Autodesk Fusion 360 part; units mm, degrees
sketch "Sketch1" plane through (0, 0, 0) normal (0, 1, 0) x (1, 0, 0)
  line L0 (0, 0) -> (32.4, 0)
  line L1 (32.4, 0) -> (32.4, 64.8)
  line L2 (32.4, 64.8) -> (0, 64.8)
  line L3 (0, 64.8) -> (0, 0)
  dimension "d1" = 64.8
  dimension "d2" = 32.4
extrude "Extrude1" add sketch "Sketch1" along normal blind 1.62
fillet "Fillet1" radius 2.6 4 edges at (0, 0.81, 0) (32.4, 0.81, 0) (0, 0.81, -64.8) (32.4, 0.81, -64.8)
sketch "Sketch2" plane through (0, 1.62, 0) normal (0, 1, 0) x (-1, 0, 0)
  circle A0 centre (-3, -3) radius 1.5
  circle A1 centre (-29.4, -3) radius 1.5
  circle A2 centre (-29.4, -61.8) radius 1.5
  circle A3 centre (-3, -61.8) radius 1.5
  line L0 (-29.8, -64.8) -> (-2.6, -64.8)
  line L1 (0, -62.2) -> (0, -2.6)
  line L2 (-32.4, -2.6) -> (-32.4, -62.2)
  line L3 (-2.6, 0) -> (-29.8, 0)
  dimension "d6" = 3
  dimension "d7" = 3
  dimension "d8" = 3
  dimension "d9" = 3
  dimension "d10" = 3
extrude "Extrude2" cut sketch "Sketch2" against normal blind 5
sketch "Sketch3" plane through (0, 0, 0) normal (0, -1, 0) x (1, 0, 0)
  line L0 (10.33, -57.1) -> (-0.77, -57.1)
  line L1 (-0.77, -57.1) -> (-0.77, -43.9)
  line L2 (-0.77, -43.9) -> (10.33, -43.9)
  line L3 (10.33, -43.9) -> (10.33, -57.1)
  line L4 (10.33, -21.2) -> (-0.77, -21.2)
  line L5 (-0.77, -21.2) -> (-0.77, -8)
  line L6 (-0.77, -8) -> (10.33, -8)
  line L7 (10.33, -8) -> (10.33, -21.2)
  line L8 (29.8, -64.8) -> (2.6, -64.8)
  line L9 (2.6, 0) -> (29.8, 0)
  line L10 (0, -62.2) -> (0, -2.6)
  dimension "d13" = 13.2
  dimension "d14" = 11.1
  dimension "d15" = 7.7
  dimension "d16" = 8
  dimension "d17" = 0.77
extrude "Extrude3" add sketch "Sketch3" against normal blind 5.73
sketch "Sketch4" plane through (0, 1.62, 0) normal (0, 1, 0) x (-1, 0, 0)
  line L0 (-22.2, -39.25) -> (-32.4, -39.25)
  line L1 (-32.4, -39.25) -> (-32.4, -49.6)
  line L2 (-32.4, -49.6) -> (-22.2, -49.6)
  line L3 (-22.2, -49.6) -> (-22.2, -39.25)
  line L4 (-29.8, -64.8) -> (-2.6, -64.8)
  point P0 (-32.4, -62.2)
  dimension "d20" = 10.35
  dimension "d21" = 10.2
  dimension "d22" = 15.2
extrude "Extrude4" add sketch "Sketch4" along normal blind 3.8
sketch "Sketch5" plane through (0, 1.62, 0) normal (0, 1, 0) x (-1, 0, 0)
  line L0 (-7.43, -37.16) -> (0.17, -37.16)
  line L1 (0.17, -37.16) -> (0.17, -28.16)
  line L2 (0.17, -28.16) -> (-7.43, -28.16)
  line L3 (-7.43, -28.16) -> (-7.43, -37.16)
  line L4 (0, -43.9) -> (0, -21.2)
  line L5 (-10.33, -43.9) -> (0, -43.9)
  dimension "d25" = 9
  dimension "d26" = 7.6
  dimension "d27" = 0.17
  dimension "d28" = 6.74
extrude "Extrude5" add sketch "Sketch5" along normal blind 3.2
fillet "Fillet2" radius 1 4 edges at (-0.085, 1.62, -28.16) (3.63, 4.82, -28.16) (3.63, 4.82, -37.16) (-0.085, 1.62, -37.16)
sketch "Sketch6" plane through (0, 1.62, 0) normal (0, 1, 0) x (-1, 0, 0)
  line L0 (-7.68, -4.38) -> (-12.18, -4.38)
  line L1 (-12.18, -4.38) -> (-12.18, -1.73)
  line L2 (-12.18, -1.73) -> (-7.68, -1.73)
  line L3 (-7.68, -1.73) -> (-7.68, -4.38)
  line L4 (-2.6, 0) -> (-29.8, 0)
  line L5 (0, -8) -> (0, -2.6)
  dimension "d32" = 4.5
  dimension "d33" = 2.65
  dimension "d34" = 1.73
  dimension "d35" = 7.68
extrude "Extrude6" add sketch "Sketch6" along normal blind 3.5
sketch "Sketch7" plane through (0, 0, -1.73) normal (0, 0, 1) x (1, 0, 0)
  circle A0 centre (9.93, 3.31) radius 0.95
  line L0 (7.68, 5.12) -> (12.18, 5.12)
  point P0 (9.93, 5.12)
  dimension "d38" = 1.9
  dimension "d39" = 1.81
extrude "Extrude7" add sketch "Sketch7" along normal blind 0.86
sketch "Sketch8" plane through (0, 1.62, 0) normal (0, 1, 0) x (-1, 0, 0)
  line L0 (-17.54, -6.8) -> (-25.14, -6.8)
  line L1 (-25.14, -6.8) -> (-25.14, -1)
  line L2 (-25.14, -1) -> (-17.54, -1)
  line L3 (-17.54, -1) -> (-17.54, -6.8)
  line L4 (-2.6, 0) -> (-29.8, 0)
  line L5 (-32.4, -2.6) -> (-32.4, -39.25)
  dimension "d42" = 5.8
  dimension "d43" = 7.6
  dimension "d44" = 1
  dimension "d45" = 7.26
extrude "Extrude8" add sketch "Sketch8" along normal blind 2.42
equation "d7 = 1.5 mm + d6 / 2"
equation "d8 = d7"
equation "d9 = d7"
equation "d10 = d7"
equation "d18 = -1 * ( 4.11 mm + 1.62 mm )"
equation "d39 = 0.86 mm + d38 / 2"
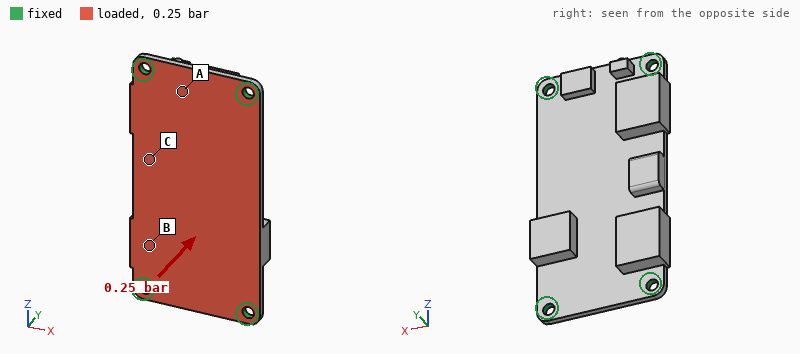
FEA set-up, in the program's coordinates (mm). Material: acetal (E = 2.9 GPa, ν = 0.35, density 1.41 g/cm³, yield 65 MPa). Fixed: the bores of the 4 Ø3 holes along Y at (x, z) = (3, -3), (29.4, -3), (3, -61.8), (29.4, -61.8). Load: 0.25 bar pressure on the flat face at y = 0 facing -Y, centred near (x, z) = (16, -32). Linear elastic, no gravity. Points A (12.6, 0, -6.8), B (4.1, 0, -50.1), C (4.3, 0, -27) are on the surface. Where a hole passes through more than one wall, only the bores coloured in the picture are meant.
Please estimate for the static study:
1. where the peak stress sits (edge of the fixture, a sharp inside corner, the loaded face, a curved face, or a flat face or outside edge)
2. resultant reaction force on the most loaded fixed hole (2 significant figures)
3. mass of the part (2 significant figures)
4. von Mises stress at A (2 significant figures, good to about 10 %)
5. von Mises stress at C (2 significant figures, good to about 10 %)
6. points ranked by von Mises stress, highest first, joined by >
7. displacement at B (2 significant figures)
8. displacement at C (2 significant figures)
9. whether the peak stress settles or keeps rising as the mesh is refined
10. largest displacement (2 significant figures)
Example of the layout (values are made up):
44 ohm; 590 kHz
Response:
edge of the fixture; 14 N; 7.5 g; 5.0 MPa; 9.6 MPa; C > A > B; 0.28 mm; 0.59 mm; keeps rising; 0.74 mm
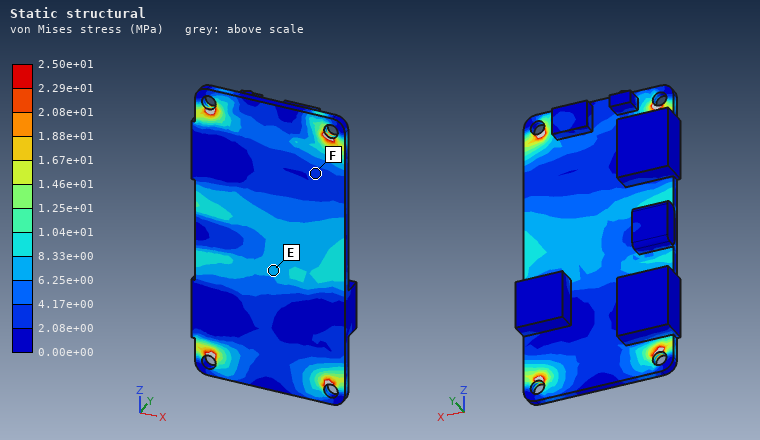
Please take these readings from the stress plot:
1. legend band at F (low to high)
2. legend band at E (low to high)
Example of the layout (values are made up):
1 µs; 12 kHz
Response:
2.08e+00 to 4.17e+00 MPa; 6.25e+00 to 8.33e+00 MPa
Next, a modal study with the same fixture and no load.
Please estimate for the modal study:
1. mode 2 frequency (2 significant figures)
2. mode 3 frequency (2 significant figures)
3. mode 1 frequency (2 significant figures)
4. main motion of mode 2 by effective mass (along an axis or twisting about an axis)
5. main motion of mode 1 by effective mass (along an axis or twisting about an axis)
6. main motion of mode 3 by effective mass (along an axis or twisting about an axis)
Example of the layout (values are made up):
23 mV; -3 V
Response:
1100 Hz; 1800 Hz; 600 Hz; twisting about Z; along Y; twisting about X
